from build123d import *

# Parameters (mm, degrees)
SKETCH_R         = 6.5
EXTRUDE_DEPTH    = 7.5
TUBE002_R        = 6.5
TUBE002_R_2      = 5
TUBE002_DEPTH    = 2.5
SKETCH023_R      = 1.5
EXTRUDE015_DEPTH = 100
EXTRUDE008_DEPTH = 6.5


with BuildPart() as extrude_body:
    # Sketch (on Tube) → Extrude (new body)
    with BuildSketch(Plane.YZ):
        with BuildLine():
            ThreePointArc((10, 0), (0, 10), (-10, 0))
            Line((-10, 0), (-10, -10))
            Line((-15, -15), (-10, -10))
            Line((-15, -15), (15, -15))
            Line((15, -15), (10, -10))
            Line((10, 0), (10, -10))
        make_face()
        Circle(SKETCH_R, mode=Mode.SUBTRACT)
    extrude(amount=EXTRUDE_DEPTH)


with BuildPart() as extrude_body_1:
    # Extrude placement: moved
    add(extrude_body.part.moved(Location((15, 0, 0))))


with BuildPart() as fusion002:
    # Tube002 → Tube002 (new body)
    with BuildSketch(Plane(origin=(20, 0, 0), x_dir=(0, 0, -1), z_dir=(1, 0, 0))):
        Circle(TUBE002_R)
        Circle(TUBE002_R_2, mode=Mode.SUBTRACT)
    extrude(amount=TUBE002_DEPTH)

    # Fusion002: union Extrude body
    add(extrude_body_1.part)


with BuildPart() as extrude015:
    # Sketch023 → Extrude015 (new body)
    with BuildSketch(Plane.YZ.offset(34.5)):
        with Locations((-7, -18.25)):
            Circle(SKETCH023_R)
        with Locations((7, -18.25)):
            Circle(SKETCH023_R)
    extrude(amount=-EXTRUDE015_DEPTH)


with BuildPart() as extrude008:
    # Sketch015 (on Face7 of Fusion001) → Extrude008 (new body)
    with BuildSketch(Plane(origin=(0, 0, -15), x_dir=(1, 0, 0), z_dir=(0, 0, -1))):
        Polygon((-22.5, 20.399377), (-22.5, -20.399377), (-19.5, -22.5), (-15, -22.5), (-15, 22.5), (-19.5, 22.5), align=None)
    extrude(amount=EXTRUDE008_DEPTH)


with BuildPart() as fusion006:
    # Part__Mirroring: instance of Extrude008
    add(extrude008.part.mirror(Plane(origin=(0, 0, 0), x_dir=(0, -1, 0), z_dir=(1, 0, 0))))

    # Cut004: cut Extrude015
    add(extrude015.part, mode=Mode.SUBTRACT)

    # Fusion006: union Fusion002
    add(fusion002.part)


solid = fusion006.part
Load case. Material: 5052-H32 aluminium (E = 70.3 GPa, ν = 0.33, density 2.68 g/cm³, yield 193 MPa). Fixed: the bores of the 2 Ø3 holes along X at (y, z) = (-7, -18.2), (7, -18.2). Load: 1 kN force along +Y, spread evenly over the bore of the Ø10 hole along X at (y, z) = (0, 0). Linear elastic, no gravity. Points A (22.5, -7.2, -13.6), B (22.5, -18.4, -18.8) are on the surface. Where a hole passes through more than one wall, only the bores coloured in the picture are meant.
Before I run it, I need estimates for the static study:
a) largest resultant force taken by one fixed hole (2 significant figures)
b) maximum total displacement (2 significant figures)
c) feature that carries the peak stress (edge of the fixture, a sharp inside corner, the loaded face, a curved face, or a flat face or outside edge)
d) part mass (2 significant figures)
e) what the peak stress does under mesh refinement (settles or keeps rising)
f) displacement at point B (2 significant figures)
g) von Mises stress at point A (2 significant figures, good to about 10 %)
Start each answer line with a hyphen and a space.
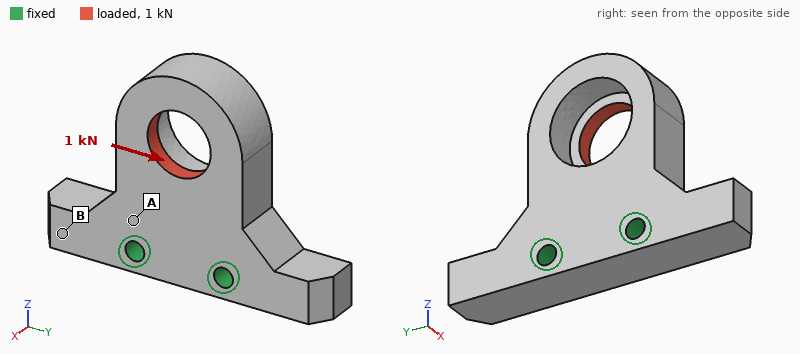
- 1.2 kN
- 28 µm
- edge of the fixture
- 13 g
- keeps rising
- 4.5 µm
- 16 MPa
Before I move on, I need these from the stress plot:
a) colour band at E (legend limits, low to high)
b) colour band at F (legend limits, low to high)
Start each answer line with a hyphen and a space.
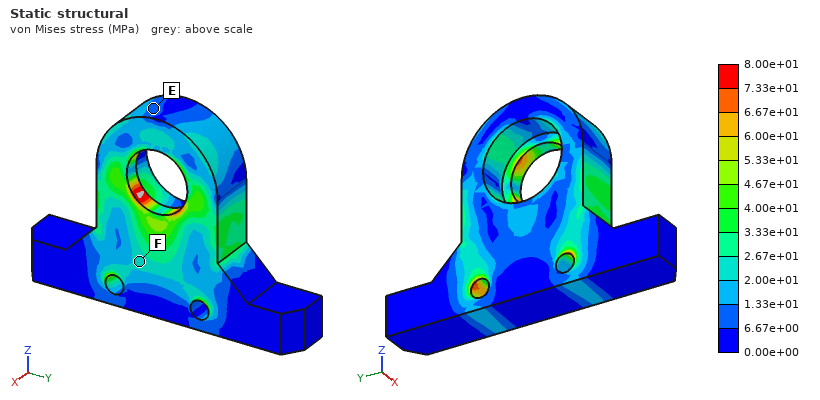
- 6.67e+00 to 1.33e+01 MPa
- 2.00e+01 to 2.67e+01 MPa
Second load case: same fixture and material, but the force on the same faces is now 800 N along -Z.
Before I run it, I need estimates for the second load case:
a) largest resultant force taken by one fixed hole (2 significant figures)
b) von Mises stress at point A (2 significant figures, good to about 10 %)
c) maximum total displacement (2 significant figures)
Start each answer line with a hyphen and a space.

- 400 N
- 18 MPa
- 18 µm
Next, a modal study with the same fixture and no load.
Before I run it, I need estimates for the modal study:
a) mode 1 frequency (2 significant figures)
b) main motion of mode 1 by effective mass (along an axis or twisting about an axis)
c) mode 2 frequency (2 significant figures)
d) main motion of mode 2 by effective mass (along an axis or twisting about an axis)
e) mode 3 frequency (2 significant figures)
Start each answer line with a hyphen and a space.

- 9500 Hz
- along X
- 16 kHz
- along Y
- 21 kHz
